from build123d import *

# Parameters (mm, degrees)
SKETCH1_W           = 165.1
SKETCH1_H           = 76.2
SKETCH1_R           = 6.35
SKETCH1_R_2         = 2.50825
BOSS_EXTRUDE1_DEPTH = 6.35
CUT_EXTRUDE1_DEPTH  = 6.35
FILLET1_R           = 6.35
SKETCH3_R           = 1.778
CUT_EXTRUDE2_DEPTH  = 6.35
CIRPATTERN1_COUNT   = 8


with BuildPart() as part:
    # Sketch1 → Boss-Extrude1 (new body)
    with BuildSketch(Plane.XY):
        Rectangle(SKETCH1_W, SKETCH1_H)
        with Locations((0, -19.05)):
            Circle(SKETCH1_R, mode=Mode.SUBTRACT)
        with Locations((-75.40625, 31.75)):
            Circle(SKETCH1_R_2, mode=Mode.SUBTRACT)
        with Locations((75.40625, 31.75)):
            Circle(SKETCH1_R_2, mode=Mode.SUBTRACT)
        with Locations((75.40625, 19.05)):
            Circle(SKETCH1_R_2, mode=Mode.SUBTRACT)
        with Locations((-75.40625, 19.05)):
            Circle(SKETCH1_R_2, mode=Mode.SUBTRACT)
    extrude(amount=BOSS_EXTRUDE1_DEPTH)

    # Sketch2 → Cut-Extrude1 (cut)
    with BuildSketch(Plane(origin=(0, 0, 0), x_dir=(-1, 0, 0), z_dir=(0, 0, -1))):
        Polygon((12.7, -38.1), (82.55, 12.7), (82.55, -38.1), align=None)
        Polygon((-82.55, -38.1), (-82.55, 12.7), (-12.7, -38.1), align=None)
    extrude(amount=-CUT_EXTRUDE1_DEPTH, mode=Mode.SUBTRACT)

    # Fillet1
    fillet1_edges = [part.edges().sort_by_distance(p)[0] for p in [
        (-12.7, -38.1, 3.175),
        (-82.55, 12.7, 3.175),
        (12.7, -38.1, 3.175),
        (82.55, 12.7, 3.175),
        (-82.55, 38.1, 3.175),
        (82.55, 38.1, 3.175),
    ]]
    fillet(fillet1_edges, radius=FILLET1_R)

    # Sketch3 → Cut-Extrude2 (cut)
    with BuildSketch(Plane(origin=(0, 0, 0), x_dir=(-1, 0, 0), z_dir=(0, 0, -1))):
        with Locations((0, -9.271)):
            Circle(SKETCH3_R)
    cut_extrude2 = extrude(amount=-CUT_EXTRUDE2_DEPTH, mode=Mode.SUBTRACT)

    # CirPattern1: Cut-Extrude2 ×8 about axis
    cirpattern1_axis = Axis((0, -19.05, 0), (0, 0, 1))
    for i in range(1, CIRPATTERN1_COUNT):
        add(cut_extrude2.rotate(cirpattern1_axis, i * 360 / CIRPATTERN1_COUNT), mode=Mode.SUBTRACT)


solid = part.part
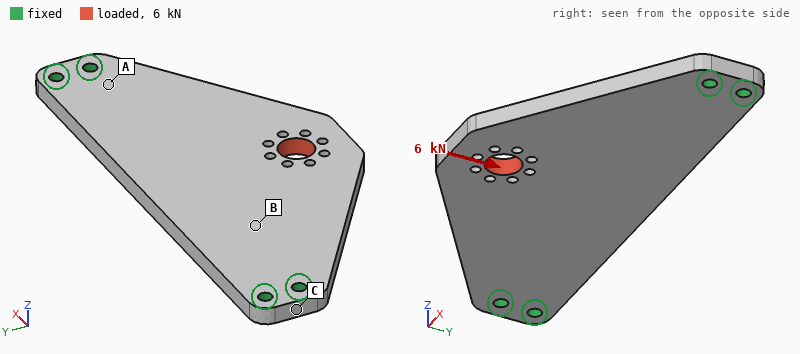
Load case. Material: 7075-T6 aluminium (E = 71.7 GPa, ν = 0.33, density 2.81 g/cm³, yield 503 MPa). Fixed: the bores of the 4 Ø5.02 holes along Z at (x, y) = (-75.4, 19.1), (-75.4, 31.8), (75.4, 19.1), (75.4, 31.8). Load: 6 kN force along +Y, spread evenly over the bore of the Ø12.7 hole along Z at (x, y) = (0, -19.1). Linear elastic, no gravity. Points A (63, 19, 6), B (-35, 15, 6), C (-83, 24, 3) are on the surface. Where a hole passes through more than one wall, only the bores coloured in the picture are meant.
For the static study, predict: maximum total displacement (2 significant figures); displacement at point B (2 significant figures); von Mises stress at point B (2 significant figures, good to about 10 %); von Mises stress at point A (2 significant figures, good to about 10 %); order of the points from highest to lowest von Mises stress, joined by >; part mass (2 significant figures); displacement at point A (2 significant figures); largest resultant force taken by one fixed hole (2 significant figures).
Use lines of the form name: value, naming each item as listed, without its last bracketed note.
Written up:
maximum total displacement: 51 µm
displacement at point B: 31 µm
von Mises stress at point B: 15 MPa
von Mises stress at point A: 27 MPa
order of the points from highest to lowest von Mises stress, joined by >: A > B > C
part mass: 160 g
displacement at point A: 9.8 µm
largest resultant force taken by one fixed hole: 3.0 kN
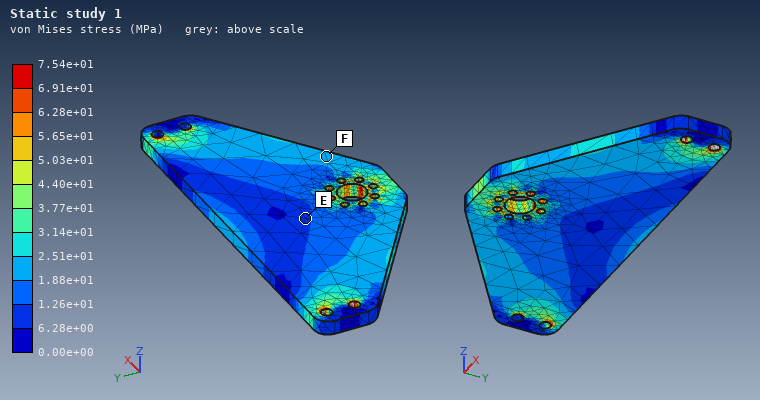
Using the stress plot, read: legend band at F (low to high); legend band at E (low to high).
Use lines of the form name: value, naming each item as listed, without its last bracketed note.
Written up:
legend band at F: 1.88e+01 to 2.51e+01 MPa
legend band at E: 6.28e+00 to 1.26e+01 MPa
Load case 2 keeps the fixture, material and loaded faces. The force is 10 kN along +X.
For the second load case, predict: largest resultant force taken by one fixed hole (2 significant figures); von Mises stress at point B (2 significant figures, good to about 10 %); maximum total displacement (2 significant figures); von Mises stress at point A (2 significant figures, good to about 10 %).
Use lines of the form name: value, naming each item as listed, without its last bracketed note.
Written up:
largest resultant force taken by one fixed hole: 3.5 kN
von Mises stress at point B: 15 MPa
maximum total displacement: 50 µm
von Mises stress at point A: 31 MPa
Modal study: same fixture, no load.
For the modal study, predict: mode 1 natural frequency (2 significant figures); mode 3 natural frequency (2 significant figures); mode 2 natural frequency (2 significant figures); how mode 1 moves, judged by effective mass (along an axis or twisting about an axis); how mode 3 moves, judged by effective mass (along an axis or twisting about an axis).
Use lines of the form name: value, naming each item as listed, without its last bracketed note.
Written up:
mode 1 natural frequency: 940 Hz
mode 3 natural frequency: 3000 Hz
mode 2 natural frequency: 1900 Hz
how mode 1 moves, judged by effective mass: along Z
how mode 3 moves, judged by effective mass: twisting about Y
